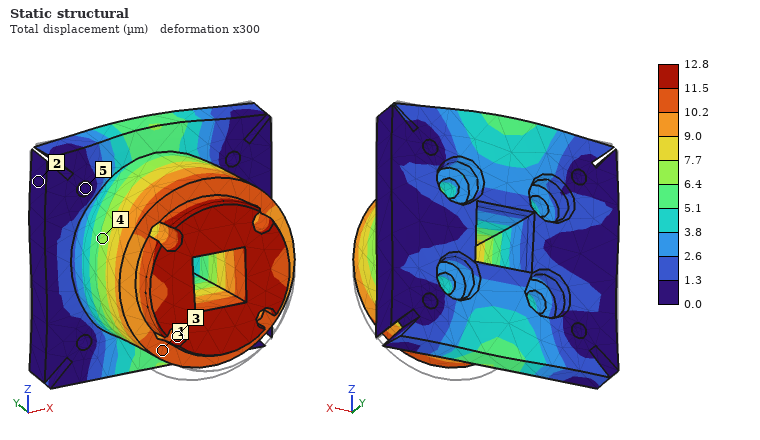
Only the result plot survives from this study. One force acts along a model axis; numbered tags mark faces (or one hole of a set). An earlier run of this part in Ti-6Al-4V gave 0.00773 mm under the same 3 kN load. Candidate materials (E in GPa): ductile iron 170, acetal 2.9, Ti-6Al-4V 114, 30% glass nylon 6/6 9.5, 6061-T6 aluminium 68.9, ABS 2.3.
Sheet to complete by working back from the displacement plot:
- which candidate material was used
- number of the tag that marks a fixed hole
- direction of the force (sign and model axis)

6061-T6 aluminium
5
+Z
